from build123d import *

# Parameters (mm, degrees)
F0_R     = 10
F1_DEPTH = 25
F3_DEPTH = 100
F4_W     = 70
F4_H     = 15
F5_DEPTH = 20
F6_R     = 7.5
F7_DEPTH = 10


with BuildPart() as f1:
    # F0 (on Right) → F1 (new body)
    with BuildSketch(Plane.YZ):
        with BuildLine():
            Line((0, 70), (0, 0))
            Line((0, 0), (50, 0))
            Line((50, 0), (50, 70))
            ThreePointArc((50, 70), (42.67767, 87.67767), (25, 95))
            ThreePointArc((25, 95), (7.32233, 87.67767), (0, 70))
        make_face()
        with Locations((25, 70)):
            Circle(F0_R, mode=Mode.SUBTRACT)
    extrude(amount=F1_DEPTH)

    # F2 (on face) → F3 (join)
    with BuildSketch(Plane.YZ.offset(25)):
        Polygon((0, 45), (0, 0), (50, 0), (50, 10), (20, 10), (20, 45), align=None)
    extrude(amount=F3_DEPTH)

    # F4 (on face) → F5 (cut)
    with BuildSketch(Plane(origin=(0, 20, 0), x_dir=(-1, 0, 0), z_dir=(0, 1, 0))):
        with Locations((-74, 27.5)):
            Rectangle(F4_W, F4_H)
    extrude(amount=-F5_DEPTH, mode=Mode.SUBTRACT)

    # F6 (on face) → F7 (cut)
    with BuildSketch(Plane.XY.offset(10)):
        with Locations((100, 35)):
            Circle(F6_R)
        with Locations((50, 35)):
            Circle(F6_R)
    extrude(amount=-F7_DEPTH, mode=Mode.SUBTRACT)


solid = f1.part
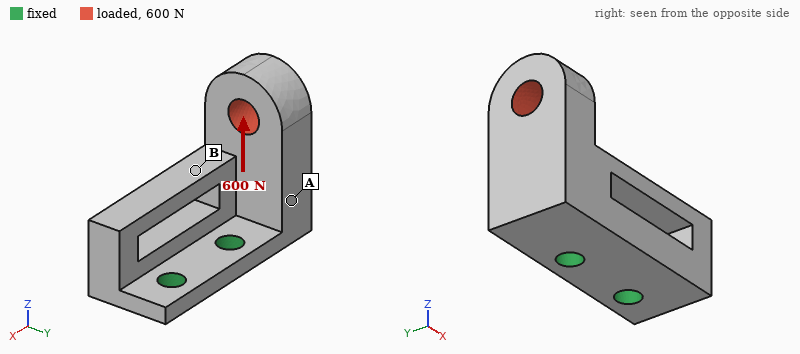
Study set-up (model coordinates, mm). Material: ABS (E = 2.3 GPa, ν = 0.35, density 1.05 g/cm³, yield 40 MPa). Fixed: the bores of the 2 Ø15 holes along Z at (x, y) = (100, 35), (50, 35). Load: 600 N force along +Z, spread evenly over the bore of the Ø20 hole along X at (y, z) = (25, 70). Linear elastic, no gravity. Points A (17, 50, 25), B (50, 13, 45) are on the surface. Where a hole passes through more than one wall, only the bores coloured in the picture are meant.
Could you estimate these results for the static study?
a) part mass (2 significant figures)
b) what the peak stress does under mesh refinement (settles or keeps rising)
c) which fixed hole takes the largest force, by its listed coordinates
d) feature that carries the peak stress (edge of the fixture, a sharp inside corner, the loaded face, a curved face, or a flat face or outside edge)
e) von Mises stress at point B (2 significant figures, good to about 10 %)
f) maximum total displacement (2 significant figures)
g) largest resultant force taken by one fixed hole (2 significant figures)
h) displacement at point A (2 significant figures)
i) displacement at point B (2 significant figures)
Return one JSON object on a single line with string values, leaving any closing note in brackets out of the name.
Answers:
{"part mass": "210 g", "what the peak stress does under mesh refinement": "keeps rising", "which fixed hole takes the largest force, by its listed coordinates": "(50, 35)", "feature that carries the peak stress": "edge of the fixture", "von Mises stress at point B": "3.1 MPa", "maximum total displacement": "0.90 mm", "largest resultant force taken by one fixed hole": "820 N", "displacement at point A": "0.29 mm", "displacement at point B": "0.29 mm"}
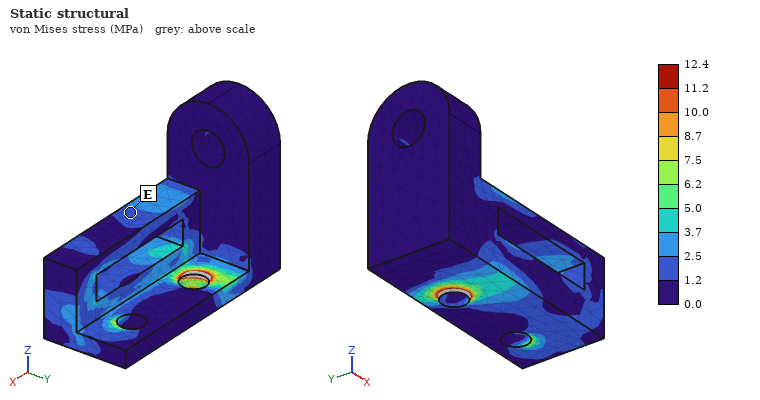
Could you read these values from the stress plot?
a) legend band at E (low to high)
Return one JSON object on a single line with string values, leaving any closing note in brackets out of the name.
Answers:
{"legend band at E": "1.2 to 2.5 MPa"}
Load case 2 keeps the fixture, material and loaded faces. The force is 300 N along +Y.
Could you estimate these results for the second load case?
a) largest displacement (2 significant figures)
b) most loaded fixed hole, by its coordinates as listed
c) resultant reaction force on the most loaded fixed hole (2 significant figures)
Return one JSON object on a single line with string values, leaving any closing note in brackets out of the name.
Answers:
{"largest displacement": "1.6 mm", "most loaded fixed hole, by its coordinates as listed": "(50, 35)", "resultant reaction force on the most loaded fixed hole": "410 N"}
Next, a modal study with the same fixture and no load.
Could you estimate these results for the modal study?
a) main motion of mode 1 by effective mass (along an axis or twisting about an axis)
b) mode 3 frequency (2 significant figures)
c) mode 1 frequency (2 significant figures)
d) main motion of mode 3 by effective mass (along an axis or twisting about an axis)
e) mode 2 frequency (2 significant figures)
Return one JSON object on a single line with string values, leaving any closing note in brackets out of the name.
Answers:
{"main motion of mode 1 by effective mass": "along Y", "mode 3 frequency": "1000 Hz", "mode 1 frequency": "300 Hz", "main motion of mode 3 by effective mass": "along Z", "mode 2 frequency": "430 Hz"}
